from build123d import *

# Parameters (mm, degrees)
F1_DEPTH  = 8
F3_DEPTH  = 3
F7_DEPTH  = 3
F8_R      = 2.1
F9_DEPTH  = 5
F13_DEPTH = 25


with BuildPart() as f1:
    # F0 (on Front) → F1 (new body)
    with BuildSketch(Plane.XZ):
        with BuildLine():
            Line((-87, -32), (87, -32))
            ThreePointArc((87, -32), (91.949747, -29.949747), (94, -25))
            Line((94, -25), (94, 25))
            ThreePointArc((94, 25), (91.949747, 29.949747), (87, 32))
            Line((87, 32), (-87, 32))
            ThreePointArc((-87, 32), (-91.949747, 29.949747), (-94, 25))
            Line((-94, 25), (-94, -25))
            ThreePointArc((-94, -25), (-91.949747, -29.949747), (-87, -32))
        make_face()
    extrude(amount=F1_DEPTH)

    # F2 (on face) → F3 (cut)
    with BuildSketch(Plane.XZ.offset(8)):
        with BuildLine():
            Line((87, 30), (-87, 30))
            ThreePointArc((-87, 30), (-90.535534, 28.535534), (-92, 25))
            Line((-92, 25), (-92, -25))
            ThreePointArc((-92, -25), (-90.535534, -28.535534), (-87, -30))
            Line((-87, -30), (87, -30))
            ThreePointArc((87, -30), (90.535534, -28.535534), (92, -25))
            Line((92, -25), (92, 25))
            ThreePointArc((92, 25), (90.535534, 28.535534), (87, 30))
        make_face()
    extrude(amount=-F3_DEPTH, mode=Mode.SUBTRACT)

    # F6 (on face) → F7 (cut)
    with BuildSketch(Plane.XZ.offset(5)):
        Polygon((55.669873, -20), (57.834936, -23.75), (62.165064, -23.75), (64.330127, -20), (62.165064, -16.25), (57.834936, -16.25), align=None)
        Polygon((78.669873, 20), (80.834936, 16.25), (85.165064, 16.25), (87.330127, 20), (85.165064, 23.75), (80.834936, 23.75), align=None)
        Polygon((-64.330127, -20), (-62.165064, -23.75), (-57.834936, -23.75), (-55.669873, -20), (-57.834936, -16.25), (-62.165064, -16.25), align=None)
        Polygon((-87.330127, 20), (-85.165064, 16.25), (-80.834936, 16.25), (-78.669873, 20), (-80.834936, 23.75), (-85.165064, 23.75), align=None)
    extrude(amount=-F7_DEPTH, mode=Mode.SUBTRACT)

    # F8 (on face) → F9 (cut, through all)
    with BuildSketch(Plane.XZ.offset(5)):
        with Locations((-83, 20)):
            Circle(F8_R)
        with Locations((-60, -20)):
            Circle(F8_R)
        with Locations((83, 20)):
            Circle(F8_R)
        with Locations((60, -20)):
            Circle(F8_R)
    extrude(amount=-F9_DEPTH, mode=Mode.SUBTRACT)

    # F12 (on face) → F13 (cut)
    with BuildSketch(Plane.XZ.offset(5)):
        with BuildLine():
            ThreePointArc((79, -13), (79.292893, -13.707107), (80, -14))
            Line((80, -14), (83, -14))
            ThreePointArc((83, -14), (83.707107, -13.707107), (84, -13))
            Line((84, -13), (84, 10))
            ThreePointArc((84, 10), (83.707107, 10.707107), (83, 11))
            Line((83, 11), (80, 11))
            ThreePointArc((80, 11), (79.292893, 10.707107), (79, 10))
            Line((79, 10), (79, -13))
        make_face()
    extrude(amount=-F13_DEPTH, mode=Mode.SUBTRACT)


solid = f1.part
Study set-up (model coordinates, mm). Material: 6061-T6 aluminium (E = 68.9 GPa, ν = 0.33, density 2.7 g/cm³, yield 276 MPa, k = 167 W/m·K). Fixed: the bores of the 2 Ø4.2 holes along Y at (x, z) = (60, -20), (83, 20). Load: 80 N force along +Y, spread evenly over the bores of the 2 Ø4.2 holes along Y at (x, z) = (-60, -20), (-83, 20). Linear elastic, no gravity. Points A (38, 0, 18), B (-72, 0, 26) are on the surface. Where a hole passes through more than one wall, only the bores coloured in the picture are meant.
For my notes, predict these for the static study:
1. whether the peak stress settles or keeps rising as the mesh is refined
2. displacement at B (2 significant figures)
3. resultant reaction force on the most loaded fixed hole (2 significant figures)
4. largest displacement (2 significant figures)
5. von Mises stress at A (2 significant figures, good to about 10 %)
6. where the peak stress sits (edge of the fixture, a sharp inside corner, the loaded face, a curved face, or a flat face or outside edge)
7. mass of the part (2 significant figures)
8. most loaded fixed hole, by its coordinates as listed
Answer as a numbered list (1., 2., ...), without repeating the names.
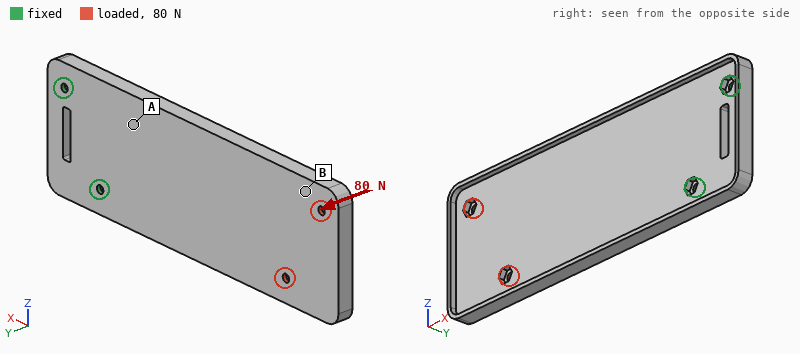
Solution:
1. keeps rising
2. 1.8 mm
3. 160 N
4. 2.2 mm
5. 24 MPa
6. edge of the fixture
7. 170 g
8. (60, -20)
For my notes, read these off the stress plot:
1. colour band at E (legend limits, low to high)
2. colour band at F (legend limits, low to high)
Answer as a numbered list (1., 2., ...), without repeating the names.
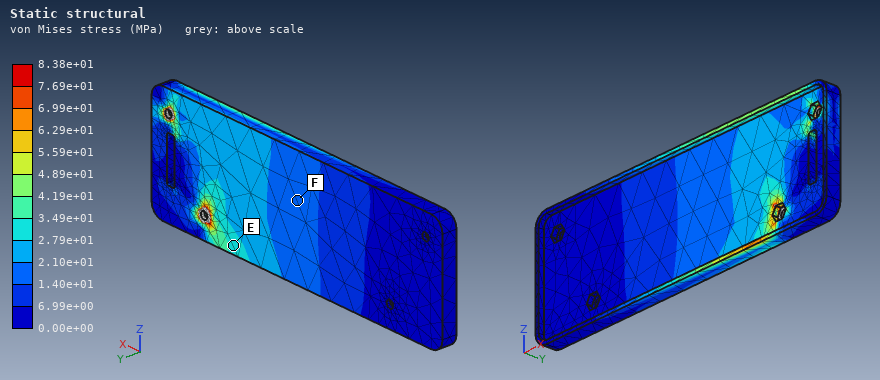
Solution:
1. 2.79e+01 to 3.49e+01 MPa
2. 1.40e+01 to 2.10e+01 MPa
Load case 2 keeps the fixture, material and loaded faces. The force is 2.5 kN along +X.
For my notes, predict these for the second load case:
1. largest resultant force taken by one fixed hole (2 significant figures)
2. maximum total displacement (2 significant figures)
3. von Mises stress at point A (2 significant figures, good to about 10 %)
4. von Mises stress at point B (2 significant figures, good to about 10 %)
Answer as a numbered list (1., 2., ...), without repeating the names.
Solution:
1. 1.3 kN
2. 0.84 mm
3. 19 MPa
4. 21 MPa
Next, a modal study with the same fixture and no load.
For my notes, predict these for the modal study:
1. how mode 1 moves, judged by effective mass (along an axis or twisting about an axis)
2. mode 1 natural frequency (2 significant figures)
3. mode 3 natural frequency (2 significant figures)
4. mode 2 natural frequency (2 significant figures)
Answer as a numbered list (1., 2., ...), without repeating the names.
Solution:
1. along Y
2. 140 Hz
3. 950 Hz
4. 700 Hz
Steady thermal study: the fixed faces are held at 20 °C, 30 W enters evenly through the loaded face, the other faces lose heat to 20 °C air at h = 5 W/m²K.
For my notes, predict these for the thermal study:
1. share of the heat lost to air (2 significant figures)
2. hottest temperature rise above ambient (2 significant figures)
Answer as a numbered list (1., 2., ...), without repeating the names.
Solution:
1. 18 %
2. 82 K
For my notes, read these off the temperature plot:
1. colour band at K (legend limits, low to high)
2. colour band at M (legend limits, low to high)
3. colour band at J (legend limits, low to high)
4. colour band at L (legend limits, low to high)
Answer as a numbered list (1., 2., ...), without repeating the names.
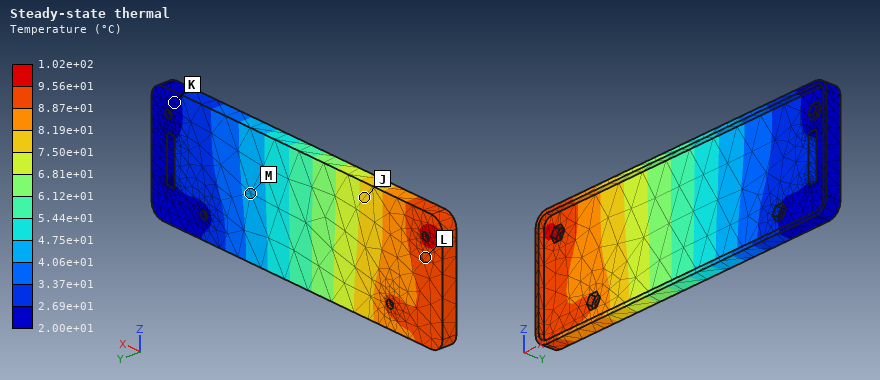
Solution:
1. 2.00e+01 to 2.69e+01 °C
2. 4.06e+01 to 4.75e+01 °C
3. 7.50e+01 to 8.19e+01 °C
4. 8.87e+01 to 9.56e+01 °C
